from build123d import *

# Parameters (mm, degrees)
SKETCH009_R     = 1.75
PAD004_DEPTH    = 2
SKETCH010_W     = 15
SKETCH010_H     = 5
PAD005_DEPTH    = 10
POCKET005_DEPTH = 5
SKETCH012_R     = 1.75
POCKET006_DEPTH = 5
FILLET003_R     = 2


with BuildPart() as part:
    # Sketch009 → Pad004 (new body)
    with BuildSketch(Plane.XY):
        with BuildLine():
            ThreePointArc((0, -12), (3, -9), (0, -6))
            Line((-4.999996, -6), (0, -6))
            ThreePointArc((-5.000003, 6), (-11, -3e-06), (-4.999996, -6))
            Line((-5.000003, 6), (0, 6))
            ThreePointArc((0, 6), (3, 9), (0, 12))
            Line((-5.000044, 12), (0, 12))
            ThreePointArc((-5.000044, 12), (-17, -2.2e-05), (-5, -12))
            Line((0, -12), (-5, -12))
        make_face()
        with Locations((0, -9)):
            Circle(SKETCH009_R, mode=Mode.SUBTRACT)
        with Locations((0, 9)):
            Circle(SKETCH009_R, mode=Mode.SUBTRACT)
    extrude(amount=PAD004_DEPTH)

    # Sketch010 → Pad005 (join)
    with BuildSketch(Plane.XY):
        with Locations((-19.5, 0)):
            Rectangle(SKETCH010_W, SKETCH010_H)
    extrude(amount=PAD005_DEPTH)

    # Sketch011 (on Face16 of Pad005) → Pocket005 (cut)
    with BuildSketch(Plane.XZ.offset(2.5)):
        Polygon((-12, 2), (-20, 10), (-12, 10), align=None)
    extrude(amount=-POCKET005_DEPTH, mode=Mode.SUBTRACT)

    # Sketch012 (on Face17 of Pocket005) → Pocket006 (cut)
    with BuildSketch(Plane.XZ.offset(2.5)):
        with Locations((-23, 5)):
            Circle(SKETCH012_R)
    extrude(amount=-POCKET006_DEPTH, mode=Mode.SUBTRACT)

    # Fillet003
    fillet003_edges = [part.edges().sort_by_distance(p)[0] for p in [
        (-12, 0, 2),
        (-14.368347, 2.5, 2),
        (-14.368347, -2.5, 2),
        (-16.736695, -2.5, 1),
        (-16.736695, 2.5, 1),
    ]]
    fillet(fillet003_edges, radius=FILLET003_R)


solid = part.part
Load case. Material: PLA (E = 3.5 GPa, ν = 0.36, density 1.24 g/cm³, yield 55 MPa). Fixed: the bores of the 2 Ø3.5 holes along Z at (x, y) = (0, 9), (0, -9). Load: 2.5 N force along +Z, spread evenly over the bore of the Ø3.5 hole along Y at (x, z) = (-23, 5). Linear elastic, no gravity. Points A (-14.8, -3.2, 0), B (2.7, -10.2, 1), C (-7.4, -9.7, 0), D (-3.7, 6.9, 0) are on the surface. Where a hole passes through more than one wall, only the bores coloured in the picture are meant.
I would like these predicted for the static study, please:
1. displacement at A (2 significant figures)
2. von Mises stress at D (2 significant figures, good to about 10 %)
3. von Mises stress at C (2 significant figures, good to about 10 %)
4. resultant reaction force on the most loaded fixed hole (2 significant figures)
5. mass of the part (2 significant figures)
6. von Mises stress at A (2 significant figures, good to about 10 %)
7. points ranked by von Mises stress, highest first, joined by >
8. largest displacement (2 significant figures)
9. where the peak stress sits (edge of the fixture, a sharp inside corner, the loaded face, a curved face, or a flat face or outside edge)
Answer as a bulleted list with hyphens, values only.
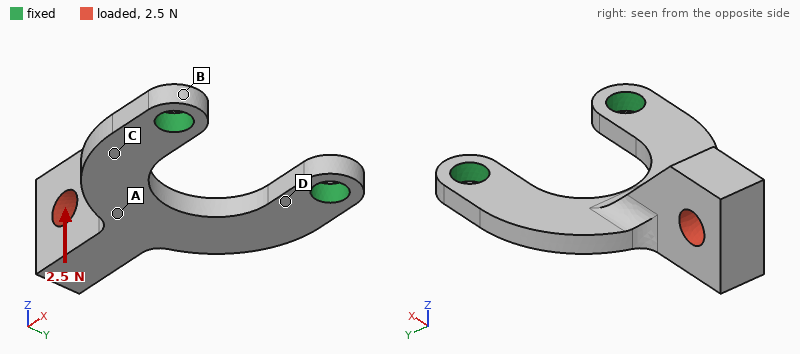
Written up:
- 0.15 mm
- 5.9 MPa
- 4.7 MPa
- 1.3 N
- 1.2 g
- 2.3 MPa
- D > C > A > B
- 0.42 mm
- a flat face or outside edge
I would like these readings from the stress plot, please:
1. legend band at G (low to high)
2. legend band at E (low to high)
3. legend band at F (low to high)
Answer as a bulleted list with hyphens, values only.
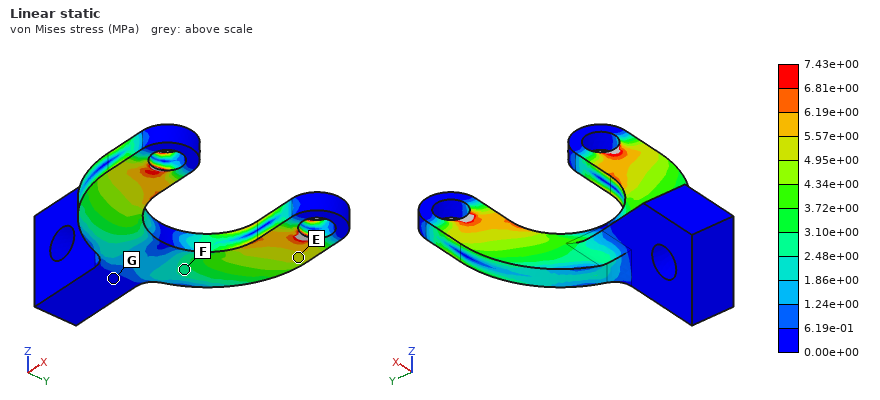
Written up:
- 0.00e+00 to 6.19e-01 MPa
- 4.95e+00 to 5.57e+00 MPa
- 2.48e+00 to 3.10e+00 MPa
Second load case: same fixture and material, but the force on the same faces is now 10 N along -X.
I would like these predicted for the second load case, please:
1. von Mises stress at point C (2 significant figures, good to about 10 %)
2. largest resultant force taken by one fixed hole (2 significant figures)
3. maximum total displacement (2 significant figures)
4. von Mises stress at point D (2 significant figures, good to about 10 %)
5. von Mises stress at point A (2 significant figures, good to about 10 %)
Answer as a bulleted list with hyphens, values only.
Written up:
- 4.5 MPa
- 5.6 N
- 0.43 mm
- 4.5 MPa
- 2.6 MPa
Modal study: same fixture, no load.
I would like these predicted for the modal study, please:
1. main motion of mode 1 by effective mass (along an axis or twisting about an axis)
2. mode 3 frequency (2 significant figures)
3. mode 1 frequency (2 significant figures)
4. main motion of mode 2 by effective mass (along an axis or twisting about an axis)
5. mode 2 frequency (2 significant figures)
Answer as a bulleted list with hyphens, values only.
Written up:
- along Z
- 3600 Hz
- 580 Hz
- along Y
- 2700 Hz
